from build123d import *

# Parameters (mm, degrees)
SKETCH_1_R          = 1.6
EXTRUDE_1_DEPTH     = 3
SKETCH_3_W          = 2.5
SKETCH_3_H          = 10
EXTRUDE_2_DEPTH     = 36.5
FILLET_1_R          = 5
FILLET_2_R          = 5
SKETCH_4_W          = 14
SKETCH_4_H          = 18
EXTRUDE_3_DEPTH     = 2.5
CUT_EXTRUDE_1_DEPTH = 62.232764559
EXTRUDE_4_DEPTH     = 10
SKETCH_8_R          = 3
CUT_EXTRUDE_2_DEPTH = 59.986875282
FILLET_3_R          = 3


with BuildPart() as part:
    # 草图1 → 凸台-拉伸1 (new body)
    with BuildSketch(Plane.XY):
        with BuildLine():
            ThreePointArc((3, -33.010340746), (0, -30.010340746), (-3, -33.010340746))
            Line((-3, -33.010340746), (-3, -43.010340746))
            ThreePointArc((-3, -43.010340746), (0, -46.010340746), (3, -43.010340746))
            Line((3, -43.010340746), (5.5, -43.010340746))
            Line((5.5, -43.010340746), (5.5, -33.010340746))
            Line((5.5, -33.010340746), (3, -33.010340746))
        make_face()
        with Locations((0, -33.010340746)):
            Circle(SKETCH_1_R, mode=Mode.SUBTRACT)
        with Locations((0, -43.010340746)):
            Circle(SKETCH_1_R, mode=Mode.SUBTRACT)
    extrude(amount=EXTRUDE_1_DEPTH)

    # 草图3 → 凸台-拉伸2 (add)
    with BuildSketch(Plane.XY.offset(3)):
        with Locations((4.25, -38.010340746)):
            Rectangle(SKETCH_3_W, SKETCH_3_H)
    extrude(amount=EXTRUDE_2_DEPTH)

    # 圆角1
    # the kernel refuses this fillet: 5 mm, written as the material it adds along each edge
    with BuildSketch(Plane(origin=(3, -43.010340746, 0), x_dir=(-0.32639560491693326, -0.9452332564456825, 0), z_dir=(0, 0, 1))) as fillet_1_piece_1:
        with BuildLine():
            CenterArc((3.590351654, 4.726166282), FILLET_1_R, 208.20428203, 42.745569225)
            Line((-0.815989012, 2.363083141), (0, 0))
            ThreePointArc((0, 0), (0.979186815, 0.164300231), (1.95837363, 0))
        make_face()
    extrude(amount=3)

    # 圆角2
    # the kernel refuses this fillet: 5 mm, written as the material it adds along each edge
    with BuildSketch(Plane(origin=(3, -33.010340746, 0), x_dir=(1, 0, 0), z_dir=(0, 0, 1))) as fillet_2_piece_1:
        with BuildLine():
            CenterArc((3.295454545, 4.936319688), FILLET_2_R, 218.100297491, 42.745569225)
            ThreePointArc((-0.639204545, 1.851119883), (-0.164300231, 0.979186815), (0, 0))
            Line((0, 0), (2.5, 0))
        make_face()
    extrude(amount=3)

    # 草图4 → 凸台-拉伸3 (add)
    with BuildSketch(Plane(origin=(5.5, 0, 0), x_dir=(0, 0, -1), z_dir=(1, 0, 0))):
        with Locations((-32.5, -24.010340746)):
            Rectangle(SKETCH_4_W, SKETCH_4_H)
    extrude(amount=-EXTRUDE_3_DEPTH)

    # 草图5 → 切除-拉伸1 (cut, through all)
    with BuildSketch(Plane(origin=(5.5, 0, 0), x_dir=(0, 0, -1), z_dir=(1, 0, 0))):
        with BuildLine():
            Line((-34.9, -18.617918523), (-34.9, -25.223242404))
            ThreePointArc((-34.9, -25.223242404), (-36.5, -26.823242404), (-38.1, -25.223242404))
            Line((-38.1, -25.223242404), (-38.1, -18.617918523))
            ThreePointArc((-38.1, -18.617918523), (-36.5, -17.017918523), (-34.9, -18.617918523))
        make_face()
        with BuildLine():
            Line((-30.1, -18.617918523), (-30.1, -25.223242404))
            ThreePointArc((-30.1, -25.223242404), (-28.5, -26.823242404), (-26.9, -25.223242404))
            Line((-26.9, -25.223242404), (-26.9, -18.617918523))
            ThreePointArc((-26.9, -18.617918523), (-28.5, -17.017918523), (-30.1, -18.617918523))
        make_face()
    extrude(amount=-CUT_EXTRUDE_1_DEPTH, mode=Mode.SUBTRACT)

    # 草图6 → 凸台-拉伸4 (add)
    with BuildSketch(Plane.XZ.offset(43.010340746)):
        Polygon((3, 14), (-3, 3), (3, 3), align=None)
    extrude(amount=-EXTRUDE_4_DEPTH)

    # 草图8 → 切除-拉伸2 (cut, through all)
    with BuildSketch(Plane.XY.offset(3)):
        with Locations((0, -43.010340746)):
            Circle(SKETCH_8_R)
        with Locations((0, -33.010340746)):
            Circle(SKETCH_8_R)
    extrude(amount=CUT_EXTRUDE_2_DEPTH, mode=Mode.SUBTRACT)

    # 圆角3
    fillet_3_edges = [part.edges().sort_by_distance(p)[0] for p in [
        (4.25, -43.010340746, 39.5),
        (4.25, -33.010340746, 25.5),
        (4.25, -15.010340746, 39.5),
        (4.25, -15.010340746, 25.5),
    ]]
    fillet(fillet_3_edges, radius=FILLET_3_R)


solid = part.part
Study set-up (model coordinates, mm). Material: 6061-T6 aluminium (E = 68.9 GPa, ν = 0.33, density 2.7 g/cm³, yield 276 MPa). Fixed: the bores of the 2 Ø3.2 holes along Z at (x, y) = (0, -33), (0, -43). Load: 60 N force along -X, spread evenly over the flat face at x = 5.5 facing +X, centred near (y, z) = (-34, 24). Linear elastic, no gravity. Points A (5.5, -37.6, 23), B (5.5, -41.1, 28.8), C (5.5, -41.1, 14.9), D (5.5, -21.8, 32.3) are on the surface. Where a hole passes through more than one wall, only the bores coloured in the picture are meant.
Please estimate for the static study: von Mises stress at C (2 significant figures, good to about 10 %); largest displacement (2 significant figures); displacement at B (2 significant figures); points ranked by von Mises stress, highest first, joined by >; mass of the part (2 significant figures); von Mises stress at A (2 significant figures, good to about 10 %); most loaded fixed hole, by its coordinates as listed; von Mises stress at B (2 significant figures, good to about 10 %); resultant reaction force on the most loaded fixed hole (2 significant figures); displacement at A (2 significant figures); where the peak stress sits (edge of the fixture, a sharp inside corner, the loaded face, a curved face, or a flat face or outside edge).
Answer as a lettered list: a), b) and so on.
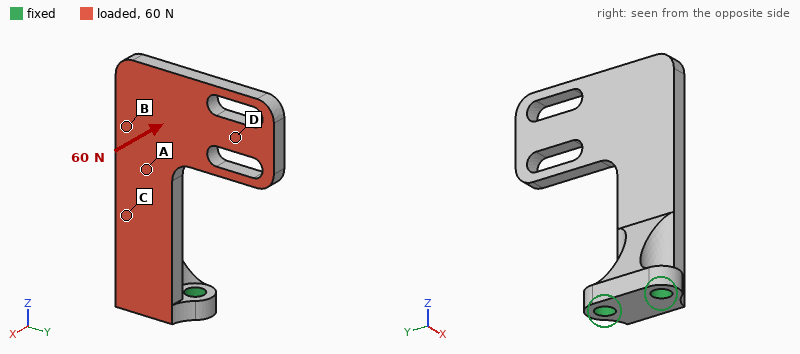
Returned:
a) 58 MPa
b) 0.33 mm
c) 0.12 mm
d) C > A > B > D
e) 5.0 g
f) 36 MPa
g) (0, -33)
h) 17 MPa
i) 55 N
j) 0.080 mm
k) a flat face or outside edge
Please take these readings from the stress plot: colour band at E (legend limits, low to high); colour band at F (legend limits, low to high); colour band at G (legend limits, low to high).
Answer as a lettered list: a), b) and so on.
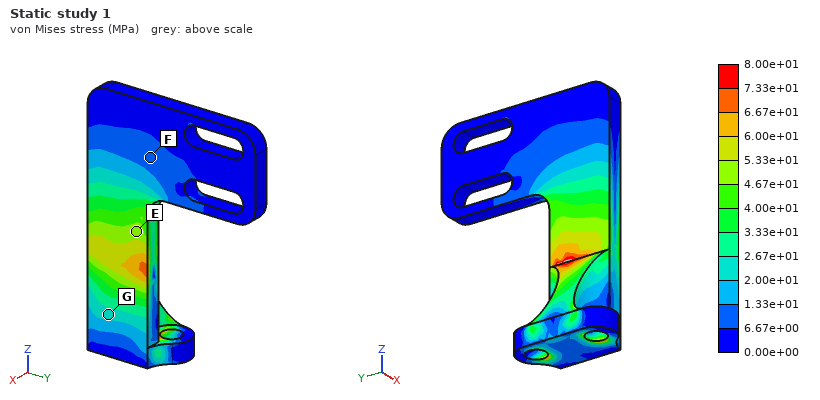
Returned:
a) 4.67e+01 to 5.33e+01 MPa
b) 6.67e+00 to 1.33e+01 MPa
c) 2.00e+01 to 2.67e+01 MPa
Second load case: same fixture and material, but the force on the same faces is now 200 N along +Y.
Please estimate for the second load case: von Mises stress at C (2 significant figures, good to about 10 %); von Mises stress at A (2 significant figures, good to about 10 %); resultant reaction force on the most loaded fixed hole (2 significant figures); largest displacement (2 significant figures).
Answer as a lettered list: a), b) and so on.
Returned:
a) 36 MPa
b) 27 MPa
c) 540 N
d) 0.19 mm
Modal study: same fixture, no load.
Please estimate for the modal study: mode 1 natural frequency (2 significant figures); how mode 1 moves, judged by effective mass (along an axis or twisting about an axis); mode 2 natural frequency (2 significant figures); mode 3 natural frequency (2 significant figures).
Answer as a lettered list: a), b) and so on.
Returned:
a) 1400 Hz
b) along X
c) 3200 Hz
d) 3300 Hz
